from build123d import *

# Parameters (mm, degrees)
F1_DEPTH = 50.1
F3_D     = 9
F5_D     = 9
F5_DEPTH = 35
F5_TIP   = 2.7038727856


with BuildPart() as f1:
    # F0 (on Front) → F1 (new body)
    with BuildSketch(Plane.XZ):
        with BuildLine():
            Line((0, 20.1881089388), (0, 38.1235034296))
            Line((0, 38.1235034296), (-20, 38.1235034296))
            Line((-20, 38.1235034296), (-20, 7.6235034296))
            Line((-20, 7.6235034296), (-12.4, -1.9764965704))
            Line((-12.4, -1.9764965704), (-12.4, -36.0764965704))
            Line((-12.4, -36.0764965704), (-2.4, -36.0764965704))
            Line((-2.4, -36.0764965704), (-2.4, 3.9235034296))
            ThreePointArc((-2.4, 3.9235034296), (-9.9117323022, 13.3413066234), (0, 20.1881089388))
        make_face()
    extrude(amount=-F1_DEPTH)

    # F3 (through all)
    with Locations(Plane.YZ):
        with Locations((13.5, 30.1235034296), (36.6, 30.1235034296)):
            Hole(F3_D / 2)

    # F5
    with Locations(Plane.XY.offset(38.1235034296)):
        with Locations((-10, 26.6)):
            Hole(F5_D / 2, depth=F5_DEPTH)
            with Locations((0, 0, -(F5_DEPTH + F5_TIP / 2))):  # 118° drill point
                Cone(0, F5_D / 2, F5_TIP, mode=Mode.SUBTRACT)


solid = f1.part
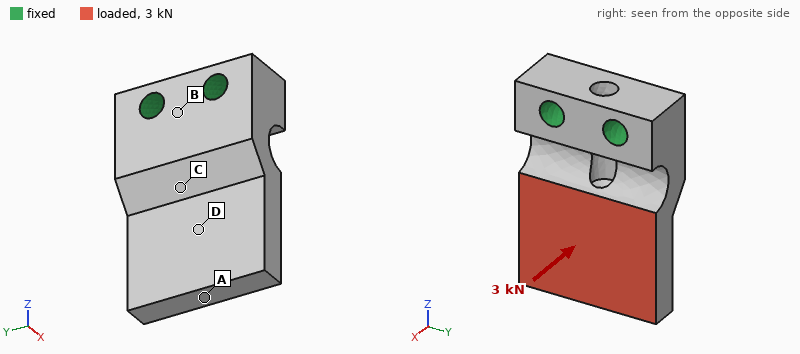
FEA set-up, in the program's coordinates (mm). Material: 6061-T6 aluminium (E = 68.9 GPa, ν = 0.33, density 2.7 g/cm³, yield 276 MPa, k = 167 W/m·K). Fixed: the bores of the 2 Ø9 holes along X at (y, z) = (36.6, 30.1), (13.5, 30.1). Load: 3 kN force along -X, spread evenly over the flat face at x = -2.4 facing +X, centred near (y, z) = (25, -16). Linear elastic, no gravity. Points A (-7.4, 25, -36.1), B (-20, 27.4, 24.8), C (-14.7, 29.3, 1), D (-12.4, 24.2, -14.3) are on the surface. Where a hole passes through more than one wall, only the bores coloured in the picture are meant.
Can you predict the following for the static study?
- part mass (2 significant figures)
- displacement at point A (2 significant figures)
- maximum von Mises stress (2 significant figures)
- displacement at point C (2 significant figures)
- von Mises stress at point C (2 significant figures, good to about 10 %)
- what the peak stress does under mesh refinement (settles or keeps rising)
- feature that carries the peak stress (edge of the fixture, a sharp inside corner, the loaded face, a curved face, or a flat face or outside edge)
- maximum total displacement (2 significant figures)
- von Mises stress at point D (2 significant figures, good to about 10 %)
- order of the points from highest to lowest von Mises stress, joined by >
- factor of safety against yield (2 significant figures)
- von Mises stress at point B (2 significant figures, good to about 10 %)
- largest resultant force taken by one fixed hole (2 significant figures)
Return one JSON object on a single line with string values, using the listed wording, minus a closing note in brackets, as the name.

{"part mass": "120 g", "displacement at point A": "0.41 mm", "maximum von Mises stress": "180 MPa", "displacement at point C": "0.082 mm", "von Mises stress at point C": "88 MPa", "what the peak stress does under mesh refinement": "settles", "feature that carries the peak stress": "a curved face", "maximum total displacement": "0.42 mm", "von Mises stress at point D": "23 MPa", "order of the points from highest to lowest von Mises stress, joined by >": "C > B > D > A", "factor of safety against yield": "1.5", "von Mises stress at point B": "47 MPa", "largest resultant force taken by one fixed hole": "1.6 kN"}
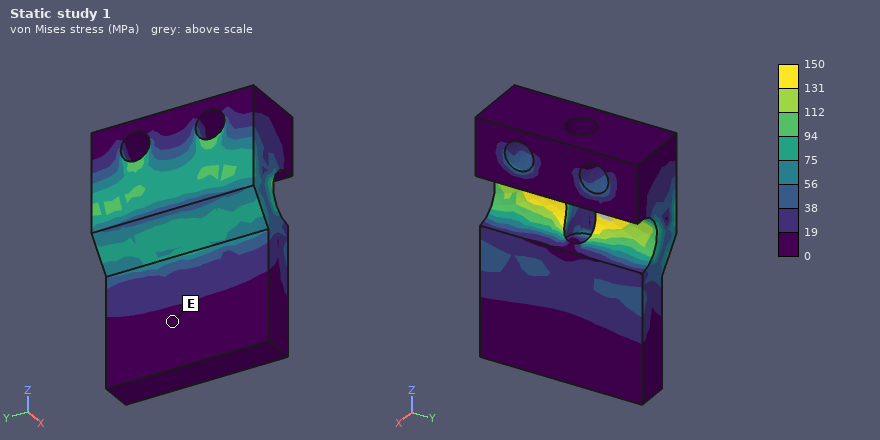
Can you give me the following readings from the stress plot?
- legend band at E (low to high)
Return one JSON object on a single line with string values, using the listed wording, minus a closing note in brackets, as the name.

{"legend band at E": "0 to 19 MPa"}
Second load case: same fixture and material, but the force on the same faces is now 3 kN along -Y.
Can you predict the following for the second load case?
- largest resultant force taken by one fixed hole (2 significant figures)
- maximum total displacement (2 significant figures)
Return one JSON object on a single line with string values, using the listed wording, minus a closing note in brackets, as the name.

{"largest resultant force taken by one fixed hole": "4.2 kN", "maximum total displacement": "59 µm"}
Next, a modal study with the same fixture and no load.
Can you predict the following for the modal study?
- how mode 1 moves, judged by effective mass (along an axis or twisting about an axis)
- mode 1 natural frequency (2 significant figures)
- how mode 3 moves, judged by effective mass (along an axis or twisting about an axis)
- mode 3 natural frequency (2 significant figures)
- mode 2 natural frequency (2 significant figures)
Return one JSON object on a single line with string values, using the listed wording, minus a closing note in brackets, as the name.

{"how mode 1 moves, judged by effective mass": "along X", "mode 1 natural frequency": "2200 Hz", "how mode 3 moves, judged by effective mass": "along Y", "mode 3 natural frequency": "6100 Hz", "mode 2 natural frequency": "5700 Hz"}
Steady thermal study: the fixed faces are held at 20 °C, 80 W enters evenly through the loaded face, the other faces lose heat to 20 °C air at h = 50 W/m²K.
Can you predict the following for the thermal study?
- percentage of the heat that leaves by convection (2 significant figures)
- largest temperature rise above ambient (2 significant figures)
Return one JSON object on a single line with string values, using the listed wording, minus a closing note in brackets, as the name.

{"percentage of the heat that leaves by convection": "9.8 %", "largest temperature rise above ambient": "41 K"}
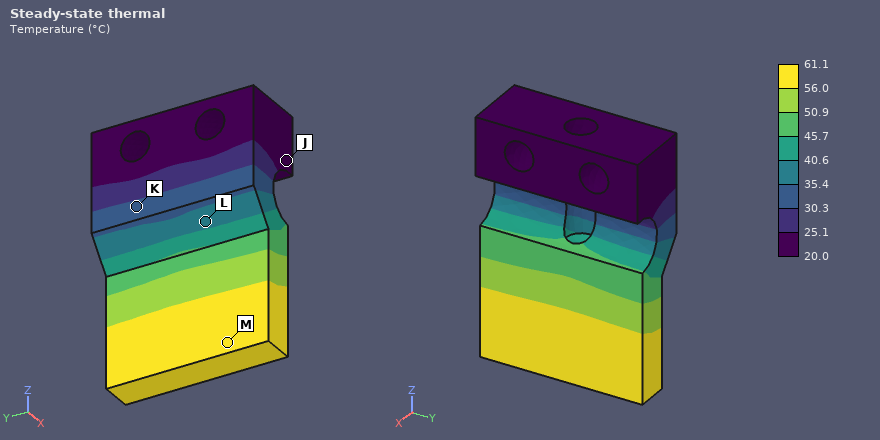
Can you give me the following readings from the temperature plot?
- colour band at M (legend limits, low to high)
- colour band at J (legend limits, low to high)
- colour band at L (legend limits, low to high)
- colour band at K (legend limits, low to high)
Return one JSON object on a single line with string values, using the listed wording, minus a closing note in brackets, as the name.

{"colour band at M": "56.0 to 61.1 °C", "colour band at J": "20.0 to 25.1 °C", "colour band at L": "35.4 to 40.6 °C", "colour band at K": "30.3 to 35.4 °C"}
